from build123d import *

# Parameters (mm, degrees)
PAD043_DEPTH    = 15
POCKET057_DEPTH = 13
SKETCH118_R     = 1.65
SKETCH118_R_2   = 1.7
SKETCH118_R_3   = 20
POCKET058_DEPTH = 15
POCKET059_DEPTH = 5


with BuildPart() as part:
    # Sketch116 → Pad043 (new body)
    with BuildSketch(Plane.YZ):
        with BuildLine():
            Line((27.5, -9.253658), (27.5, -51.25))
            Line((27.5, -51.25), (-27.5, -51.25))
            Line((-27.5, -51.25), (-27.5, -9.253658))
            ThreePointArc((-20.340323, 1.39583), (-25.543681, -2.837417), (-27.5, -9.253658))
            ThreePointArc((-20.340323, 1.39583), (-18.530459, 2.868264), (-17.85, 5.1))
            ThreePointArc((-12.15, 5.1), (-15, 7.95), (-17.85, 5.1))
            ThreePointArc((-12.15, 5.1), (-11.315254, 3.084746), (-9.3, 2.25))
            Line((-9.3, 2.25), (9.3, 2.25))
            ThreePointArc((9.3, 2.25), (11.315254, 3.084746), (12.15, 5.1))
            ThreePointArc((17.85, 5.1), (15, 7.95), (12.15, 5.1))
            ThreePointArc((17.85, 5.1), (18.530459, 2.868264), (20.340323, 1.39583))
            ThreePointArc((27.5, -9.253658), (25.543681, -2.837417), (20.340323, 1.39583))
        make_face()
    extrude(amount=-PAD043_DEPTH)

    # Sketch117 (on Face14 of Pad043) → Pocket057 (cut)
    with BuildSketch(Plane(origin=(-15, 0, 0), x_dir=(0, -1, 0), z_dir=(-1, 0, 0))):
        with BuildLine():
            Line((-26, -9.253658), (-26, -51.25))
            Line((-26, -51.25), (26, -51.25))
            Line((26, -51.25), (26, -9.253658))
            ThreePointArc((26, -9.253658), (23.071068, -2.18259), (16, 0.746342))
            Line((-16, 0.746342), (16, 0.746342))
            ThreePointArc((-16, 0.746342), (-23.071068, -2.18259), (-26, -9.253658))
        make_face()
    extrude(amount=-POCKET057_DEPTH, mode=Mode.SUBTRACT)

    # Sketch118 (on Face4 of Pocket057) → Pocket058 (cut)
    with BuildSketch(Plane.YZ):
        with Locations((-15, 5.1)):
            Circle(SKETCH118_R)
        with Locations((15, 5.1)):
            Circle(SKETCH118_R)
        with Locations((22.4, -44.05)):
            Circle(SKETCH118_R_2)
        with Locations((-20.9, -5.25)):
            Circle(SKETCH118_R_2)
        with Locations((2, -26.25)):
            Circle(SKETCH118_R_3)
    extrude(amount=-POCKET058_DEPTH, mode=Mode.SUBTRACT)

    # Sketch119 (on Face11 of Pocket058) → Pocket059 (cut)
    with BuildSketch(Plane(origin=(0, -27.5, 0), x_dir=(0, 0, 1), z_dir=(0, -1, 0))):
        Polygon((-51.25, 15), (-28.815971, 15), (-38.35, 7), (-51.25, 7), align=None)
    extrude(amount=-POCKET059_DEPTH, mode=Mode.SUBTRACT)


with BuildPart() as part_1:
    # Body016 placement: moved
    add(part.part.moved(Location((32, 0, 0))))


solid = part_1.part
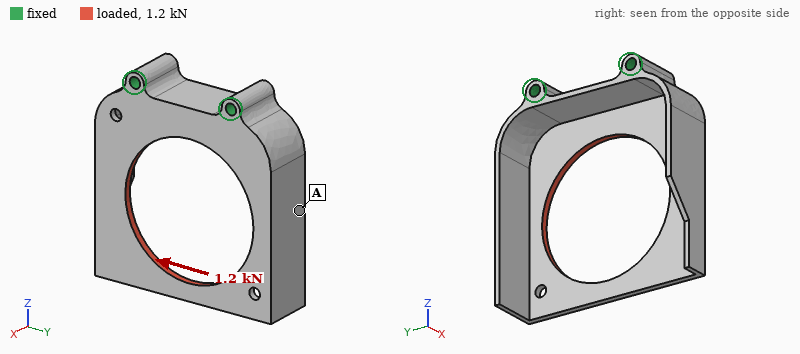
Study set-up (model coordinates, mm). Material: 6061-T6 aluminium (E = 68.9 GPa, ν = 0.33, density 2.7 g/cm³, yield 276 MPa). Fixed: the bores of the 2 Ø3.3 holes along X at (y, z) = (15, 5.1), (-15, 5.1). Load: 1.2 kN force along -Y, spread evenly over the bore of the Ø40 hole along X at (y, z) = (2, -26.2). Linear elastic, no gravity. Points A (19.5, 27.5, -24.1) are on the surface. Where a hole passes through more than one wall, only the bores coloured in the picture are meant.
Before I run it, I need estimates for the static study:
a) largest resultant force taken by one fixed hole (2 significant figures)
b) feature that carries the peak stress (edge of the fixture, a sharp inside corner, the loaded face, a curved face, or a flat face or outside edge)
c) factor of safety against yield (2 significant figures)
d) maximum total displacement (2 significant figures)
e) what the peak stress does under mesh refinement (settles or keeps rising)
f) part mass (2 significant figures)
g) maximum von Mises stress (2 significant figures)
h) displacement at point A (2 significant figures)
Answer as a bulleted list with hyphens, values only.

- 1.2 kN
- the loaded face
- 1.4
- 0.40 mm
- settles
- 18 g
- 190 MPa
- 0.20 mm
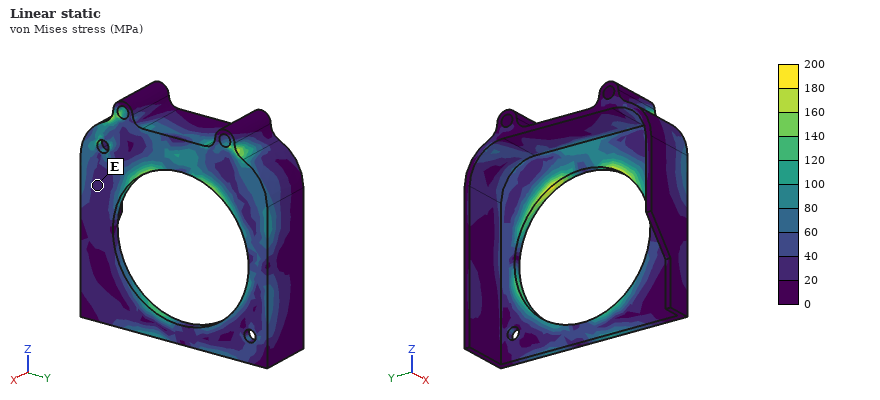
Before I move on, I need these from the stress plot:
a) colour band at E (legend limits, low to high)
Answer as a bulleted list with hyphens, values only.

- 20 to 40 MPa
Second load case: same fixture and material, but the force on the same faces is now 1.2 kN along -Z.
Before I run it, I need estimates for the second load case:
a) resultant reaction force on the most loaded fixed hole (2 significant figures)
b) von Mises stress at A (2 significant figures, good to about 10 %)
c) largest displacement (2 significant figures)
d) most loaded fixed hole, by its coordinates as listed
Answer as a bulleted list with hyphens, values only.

- 690 N
- 9.9 MPa
- 96 µm
- (15, 5.1)
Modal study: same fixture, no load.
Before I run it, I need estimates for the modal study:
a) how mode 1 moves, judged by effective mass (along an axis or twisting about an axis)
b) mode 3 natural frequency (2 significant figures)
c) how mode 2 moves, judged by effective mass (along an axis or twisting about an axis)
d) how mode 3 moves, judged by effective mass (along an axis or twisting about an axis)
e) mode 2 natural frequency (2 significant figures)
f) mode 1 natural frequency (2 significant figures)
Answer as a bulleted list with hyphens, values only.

- along X
- 2800 Hz
- twisting about Z
- along Y
- 1800 Hz
- 1200 Hz
